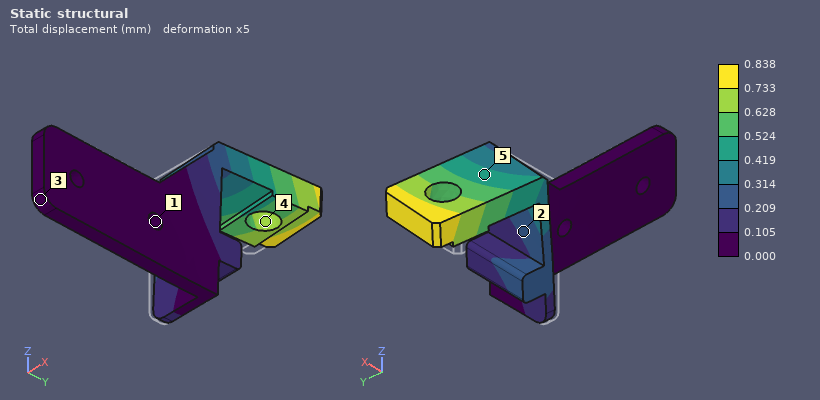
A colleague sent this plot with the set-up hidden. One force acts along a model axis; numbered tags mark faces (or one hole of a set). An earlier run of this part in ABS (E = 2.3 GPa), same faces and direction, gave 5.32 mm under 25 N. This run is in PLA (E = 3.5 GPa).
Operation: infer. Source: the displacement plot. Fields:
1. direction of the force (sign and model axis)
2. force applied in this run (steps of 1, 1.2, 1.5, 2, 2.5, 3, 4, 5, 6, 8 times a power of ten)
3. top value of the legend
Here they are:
+X
6 N
0.838 mm
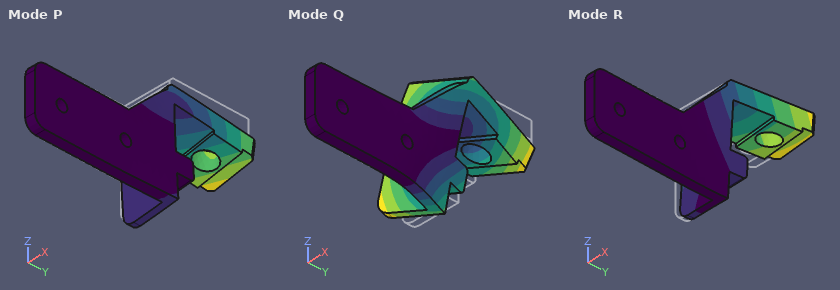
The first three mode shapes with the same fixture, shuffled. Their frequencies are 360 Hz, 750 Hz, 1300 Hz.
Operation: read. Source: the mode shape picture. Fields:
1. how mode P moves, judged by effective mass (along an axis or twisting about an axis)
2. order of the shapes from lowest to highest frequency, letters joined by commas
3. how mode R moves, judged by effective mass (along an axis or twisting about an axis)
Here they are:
along Z
R, P, Q
along X
